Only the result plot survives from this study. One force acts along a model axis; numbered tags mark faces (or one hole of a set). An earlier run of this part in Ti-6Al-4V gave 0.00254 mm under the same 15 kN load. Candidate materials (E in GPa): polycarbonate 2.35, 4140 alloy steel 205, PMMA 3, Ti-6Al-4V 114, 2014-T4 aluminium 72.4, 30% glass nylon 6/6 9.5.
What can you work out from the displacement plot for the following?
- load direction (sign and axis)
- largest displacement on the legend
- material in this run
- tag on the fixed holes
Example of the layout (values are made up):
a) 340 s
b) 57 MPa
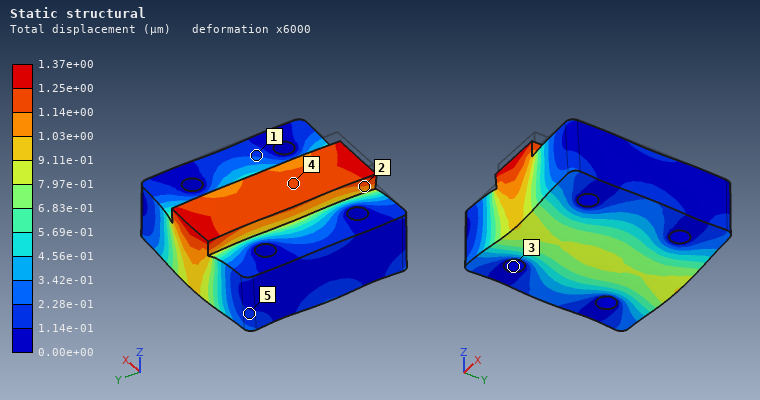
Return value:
a) -Z
b) 1.37e+00 µm
c) 4140 alloy steel
d) 3
